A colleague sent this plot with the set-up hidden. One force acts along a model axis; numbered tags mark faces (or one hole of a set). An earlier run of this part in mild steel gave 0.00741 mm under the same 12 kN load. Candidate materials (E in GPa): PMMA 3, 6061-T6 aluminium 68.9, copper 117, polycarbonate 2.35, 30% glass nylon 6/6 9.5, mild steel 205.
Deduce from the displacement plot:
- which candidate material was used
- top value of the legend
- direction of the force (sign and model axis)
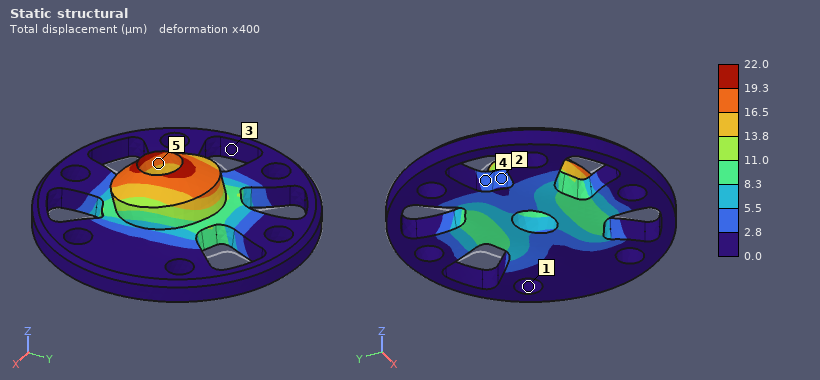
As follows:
6061-T6 aluminium
22.0 µm
-Y
